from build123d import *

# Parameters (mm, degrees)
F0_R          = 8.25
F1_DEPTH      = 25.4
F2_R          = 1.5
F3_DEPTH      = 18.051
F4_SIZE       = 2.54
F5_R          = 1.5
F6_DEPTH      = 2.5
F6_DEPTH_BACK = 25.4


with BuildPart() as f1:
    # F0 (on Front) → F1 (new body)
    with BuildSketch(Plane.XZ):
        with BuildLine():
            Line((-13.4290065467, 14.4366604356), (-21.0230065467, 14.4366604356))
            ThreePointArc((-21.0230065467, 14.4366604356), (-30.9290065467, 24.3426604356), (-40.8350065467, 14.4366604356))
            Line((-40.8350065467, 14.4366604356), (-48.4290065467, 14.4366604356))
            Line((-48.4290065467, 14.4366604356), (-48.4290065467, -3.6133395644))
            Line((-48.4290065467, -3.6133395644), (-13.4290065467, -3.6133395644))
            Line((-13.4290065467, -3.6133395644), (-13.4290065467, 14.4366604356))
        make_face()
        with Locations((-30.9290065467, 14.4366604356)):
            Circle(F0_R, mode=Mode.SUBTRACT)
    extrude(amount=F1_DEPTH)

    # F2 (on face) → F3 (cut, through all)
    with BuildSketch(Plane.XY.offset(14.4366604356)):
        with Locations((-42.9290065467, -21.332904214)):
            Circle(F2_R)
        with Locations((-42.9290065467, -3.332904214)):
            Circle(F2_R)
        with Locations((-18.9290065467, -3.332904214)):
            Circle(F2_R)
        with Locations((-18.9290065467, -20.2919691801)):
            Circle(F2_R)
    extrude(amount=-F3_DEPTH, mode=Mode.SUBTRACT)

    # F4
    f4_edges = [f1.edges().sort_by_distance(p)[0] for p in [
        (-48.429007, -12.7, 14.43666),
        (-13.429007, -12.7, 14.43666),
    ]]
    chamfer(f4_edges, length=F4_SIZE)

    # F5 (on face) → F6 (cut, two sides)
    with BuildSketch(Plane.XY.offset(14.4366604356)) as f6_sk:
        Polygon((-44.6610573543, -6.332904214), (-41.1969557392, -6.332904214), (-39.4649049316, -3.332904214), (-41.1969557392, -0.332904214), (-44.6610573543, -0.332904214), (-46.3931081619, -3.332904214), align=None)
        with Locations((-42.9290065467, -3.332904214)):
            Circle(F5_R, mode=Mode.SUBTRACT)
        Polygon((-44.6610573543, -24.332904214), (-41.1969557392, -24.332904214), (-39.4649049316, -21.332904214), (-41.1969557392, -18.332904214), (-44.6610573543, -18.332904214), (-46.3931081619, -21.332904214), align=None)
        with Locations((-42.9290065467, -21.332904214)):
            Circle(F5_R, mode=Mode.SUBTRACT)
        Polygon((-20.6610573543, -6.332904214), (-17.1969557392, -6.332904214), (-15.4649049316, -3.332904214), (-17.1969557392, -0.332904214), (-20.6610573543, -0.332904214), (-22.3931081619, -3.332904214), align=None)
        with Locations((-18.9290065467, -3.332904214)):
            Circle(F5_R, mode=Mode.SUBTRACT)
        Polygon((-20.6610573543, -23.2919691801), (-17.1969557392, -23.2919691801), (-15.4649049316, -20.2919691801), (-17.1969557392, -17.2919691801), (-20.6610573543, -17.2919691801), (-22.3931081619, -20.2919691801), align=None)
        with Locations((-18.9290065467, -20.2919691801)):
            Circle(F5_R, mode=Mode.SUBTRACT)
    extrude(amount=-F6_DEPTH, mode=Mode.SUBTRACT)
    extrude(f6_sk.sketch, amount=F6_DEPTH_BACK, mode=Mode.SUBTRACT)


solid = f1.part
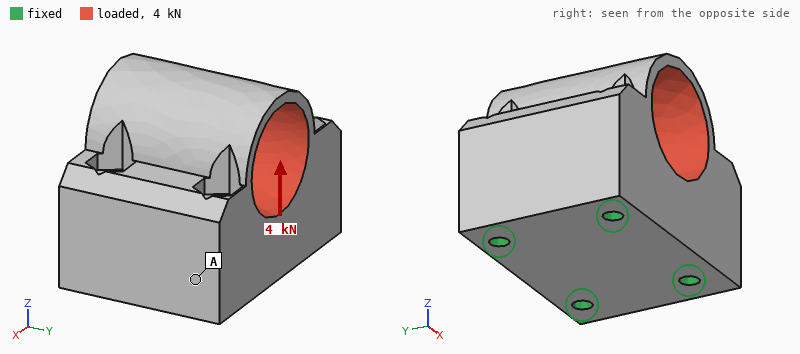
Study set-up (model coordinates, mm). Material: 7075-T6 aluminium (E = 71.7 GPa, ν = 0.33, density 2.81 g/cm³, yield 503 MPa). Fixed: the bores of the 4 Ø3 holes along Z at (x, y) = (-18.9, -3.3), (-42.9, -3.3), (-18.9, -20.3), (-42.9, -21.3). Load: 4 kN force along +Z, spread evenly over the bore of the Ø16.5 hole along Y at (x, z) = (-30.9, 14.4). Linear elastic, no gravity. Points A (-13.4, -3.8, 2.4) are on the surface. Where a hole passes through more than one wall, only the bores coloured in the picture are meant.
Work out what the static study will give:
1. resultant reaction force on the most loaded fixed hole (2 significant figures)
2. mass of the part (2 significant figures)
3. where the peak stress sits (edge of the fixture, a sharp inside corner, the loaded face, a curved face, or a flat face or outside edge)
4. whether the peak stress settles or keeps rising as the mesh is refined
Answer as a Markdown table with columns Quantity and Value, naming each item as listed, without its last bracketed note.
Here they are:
| Quantity | Value |
|---|---|
| resultant reaction force on the most loaded fixed hole | 1.1 kN |
| mass of the part | 38 g |
| where the peak stress sits | a sharp inside corner |
| whether the peak stress settles or keeps rising as the mesh is refined | keeps rising |
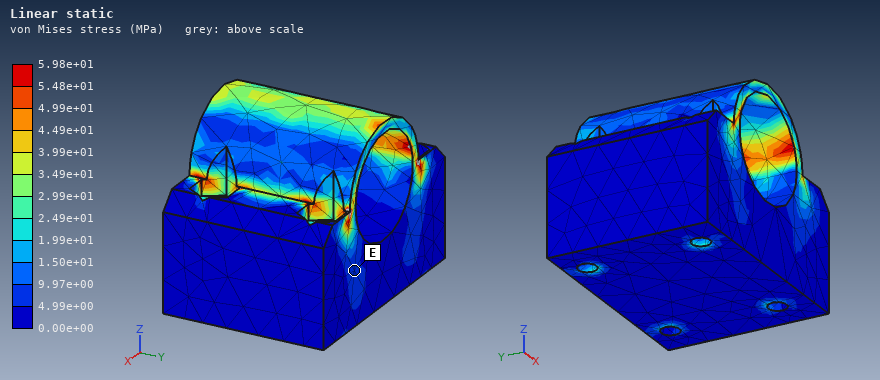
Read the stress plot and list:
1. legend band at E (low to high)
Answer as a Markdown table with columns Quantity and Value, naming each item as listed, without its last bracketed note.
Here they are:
| Quantity | Value |
|---|---|
| legend band at E | 4.99e+00 to 9.97e+00 MPa |
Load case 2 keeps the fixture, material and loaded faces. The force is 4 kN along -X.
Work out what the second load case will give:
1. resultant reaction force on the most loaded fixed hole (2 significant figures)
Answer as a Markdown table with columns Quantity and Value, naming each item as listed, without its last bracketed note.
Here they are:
| Quantity | Value |
|---|---|
| resultant reaction force on the most loaded fixed hole | 1.2 kN |
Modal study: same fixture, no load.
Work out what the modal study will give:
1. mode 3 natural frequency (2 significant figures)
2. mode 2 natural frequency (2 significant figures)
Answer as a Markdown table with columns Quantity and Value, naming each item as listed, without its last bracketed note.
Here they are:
| Quantity | Value |
|---|---|
| mode 3 natural frequency | 28 kHz |
| mode 2 natural frequency | 28 kHz |
